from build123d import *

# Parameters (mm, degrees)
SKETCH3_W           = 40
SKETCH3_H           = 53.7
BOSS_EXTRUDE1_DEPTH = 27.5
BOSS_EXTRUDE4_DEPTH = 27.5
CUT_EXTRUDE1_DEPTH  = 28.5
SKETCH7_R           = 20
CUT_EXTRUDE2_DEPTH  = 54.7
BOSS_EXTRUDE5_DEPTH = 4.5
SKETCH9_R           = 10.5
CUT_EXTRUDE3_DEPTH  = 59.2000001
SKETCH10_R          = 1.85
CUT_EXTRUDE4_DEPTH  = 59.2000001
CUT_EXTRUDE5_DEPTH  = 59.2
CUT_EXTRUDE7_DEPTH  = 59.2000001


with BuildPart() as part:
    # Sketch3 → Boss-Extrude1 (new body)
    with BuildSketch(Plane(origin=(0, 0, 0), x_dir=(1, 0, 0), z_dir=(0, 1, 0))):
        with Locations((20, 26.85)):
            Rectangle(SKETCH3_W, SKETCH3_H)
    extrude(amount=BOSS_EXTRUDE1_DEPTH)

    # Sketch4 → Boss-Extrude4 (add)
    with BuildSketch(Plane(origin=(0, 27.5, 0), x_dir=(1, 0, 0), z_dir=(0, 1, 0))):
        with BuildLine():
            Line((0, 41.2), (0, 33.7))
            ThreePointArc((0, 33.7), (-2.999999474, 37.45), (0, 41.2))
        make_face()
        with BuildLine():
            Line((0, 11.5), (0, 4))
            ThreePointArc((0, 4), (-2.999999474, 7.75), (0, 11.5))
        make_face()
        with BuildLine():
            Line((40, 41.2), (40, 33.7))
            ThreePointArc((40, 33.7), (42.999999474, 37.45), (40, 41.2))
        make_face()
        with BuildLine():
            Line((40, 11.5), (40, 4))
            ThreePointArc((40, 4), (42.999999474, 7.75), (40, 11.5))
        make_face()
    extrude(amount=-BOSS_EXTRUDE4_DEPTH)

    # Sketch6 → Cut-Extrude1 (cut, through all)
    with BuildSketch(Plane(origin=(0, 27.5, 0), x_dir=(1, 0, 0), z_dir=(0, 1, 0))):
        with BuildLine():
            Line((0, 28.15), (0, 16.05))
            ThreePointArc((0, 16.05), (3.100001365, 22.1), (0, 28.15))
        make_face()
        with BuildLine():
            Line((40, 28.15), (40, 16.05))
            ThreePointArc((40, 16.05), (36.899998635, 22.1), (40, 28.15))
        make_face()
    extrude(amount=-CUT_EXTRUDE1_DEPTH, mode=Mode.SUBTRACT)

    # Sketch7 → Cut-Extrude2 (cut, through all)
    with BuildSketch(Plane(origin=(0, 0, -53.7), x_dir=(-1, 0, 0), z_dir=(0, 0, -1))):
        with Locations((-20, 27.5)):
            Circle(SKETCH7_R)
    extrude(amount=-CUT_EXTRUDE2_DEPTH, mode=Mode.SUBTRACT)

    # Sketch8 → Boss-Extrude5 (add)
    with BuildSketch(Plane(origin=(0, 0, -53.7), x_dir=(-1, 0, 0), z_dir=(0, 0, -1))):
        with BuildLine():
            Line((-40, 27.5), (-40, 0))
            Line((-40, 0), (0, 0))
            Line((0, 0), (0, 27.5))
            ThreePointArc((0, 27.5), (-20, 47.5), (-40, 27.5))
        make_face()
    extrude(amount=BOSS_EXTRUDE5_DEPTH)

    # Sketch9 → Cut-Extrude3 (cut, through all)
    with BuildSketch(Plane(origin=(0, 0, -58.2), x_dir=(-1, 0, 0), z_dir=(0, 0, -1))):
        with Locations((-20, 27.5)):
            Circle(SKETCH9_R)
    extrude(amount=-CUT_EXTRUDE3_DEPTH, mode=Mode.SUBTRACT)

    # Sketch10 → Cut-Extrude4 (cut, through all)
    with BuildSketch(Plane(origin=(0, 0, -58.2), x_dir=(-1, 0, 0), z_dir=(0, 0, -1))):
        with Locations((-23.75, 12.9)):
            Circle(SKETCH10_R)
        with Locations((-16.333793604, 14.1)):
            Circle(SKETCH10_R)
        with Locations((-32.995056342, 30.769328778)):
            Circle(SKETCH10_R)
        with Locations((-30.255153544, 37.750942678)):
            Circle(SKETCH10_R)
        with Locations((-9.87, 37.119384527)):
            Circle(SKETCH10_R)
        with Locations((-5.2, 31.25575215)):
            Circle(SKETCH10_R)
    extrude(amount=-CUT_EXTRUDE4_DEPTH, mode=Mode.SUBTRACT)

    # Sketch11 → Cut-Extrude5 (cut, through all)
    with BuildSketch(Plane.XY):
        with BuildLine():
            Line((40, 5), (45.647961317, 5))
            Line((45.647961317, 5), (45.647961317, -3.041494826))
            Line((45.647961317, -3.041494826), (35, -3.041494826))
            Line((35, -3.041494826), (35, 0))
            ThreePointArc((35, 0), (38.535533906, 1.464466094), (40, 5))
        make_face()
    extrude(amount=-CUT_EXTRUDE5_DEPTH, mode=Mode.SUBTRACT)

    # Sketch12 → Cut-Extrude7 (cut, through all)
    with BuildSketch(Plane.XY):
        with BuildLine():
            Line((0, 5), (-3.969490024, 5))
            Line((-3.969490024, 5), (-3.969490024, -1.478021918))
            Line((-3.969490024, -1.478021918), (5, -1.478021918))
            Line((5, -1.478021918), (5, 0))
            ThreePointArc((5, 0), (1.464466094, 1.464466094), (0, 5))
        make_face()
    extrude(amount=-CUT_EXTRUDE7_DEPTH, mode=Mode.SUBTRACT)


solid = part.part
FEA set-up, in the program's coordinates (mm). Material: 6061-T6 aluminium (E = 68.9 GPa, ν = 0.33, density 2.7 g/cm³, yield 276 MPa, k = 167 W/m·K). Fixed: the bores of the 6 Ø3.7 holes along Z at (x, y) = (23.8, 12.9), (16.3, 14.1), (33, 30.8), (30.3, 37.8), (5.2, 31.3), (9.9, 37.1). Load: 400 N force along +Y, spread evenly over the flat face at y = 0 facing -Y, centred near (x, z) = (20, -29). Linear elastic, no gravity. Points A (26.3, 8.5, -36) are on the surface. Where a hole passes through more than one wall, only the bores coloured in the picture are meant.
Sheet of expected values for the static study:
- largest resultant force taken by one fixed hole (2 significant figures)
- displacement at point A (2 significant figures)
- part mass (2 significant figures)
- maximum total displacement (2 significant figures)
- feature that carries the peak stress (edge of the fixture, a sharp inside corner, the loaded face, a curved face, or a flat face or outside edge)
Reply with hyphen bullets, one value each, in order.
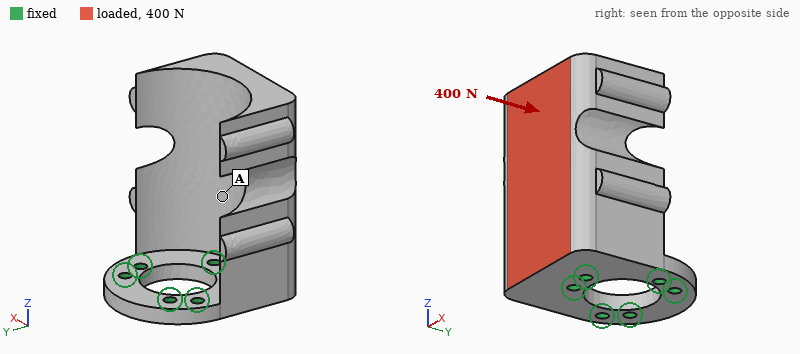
- 320 N
- 27 µm
- 84 g
- 82 µm
- a curved face
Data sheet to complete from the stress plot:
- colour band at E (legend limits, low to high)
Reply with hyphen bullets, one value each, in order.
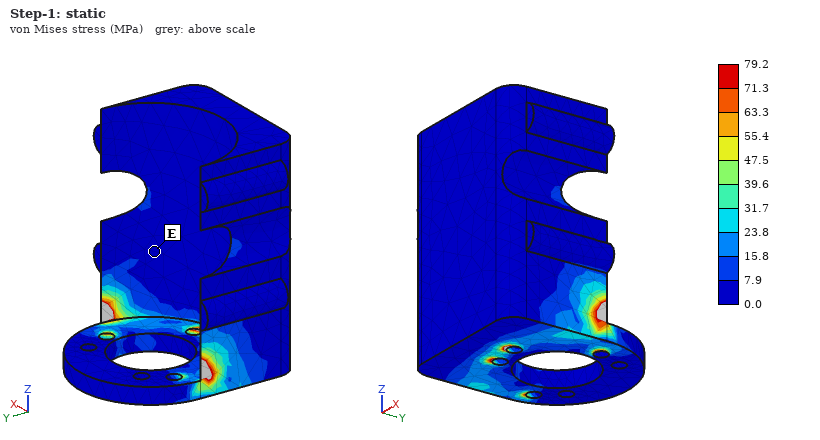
- 0.0 to 7.9 MPa
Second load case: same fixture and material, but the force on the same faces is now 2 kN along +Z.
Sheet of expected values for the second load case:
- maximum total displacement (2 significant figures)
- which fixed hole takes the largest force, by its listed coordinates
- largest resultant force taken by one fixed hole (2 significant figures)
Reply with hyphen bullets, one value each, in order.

- 0.18 mm
- (23.8, 12.9)
- 1.7 kN
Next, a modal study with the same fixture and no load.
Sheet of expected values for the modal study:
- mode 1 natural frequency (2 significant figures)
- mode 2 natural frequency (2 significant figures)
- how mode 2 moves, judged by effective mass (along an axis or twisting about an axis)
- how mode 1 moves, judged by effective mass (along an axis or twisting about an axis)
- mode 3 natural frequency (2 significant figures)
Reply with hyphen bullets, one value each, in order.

- 1600 Hz
- 1900 Hz
- along X
- along Y
- 5100 Hz
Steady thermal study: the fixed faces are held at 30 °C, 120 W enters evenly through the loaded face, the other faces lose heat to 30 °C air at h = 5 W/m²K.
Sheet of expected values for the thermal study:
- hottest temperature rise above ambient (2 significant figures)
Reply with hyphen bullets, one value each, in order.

- 76 K
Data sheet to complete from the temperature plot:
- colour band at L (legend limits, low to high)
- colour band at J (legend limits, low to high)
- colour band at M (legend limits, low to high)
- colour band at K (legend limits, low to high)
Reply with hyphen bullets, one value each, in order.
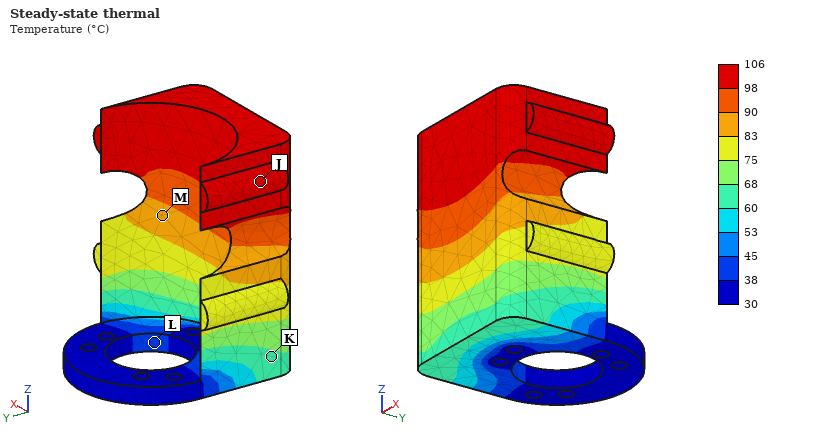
- 38 to 45 °C
- 98 to 106 °C
- 83 to 90 °C
- 60 to 68 °C
